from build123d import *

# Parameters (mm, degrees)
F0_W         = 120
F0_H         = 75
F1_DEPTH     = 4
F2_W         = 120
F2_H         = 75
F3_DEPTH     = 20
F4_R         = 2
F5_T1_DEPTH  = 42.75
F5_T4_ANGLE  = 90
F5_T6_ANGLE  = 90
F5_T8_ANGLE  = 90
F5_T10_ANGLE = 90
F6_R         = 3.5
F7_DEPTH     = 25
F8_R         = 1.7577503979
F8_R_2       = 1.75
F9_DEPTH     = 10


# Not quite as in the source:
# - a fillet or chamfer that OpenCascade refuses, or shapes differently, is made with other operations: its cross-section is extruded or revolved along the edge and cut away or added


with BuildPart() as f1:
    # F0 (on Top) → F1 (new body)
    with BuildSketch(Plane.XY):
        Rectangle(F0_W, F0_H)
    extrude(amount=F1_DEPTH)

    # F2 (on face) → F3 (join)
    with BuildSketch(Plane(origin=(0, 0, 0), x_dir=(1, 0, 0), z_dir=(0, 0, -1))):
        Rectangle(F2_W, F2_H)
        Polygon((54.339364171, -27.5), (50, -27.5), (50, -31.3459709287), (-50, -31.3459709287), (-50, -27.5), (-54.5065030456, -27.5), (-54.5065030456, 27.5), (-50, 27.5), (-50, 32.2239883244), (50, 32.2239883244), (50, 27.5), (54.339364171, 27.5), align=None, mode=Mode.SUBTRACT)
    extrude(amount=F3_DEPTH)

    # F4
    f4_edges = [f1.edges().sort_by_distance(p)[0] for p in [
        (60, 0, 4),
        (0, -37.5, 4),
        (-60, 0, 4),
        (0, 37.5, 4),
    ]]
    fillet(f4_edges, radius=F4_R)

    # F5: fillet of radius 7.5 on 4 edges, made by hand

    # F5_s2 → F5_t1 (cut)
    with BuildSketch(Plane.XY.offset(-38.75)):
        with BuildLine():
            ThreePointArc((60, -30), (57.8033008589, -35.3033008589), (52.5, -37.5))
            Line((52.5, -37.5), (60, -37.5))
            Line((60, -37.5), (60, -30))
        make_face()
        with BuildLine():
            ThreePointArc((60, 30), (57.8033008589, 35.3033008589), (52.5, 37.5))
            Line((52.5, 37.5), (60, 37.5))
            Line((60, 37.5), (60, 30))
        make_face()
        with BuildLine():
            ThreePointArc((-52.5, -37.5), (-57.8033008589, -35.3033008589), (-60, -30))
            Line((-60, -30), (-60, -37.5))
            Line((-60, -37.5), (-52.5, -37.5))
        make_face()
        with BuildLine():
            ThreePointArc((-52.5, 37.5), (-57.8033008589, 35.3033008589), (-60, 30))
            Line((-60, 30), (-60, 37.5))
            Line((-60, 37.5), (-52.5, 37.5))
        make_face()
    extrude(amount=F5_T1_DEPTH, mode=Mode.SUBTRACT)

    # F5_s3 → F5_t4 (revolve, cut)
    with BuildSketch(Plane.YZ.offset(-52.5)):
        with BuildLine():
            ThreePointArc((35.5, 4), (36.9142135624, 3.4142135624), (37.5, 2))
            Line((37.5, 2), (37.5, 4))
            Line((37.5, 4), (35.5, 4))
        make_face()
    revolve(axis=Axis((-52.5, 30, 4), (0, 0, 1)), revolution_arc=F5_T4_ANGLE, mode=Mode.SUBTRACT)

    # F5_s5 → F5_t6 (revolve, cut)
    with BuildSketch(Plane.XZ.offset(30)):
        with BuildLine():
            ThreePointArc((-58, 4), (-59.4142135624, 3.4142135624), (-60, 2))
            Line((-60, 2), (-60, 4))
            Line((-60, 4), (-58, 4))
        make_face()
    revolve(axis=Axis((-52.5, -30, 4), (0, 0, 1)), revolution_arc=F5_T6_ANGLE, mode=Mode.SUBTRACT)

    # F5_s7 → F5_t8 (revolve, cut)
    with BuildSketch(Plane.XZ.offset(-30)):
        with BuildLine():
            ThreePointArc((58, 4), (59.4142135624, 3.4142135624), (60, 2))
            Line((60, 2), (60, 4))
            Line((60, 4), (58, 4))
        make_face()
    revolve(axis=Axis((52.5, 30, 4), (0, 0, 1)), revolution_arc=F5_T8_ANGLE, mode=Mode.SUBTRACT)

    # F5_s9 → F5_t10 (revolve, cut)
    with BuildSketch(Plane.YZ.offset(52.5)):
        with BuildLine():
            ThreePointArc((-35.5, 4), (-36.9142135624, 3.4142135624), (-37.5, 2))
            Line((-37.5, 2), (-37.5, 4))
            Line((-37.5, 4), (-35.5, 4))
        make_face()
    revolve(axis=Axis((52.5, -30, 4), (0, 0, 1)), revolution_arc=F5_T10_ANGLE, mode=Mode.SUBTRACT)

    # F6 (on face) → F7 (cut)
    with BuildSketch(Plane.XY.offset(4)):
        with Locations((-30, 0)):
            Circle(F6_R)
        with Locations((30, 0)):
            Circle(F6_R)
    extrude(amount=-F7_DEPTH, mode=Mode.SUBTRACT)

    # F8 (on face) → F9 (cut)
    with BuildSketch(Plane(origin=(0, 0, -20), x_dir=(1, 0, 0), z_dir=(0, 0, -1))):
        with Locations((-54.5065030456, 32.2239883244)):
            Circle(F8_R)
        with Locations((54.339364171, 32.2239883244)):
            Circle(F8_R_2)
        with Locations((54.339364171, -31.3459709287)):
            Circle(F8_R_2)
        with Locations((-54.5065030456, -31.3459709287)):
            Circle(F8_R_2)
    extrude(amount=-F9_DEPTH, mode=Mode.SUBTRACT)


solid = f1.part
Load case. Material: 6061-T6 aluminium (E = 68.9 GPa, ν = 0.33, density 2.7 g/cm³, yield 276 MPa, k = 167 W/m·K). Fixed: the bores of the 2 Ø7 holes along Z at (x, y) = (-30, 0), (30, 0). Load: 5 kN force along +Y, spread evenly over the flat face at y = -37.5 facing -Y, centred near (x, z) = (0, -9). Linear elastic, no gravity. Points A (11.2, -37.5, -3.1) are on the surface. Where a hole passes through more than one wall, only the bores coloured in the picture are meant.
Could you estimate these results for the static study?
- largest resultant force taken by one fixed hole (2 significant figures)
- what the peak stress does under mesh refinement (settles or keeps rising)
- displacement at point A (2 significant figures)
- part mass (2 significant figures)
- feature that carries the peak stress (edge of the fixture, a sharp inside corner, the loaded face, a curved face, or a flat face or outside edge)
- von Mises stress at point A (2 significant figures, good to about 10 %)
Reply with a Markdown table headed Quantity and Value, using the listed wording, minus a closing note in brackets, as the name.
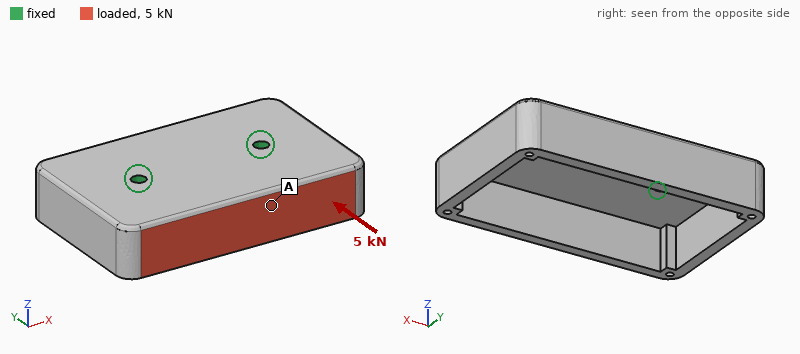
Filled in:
| Quantity | Value |
|---|---|
| largest resultant force taken by one fixed hole | 2.6 kN |
| what the peak stress does under mesh refinement | keeps rising |
| displacement at point A | 0.46 mm |
| part mass | 210 g |
| feature that carries the peak stress | edge of the fixture |
| von Mises stress at point A | 37 MPa |
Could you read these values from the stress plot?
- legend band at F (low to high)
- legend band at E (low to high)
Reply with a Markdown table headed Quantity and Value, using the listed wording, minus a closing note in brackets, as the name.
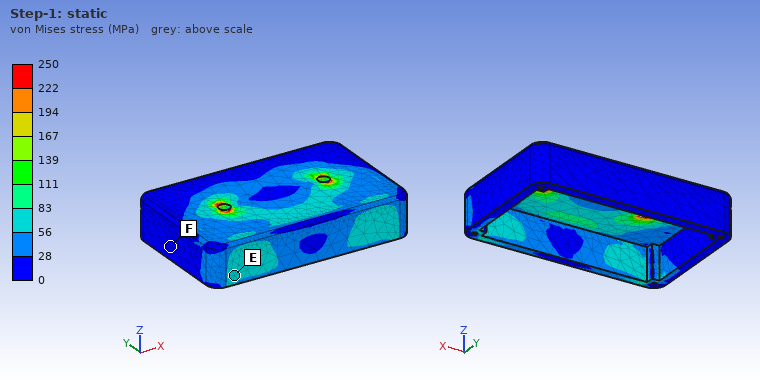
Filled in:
| Quantity | Value |
|---|---|
| legend band at F | 0 to 28 MPa |
| legend band at E | 56 to 83 MPa |
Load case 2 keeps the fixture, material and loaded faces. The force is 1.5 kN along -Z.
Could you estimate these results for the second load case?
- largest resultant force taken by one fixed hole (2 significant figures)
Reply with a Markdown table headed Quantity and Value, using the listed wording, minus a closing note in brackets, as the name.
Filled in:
| Quantity | Value |
|---|---|
| largest resultant force taken by one fixed hole | 770 N |
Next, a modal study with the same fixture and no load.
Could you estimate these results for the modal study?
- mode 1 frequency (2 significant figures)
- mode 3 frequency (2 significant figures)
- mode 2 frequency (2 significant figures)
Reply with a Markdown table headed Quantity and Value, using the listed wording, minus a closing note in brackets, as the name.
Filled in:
| Quantity | Value |
|---|---|
| mode 1 frequency | 970 Hz |
| mode 3 frequency | 1800 Hz |
| mode 2 frequency | 1600 Hz |
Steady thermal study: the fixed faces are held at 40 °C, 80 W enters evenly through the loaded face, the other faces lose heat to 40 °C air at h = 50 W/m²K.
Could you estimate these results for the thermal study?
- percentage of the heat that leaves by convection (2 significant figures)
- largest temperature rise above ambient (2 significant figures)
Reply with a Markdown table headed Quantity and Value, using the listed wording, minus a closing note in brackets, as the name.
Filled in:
| Quantity | Value |
|---|---|
| percentage of the heat that leaves by convection | 29 % |
| largest temperature rise above ambient | 40 K |
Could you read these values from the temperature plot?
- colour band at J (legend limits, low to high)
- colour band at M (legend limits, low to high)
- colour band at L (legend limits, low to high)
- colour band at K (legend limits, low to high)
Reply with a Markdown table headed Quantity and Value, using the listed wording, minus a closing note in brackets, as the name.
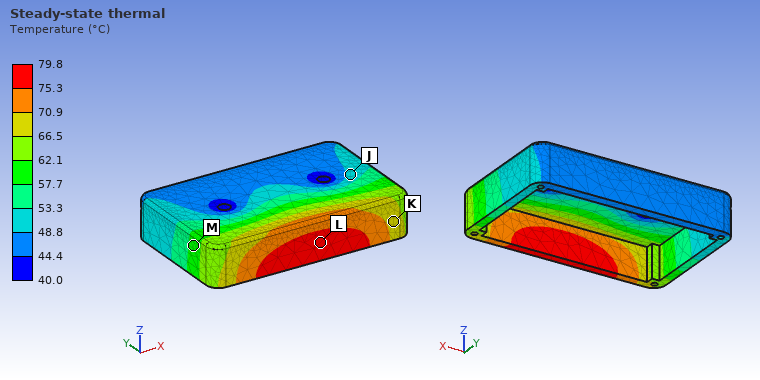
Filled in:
| Quantity | Value |
|---|---|
| colour band at J | 48.8 to 53.3 °C |
| colour band at M | 57.7 to 62.1 °C |
| colour band at L | 75.3 to 79.8 °C |
| colour band at K | 66.5 to 70.9 °C |
